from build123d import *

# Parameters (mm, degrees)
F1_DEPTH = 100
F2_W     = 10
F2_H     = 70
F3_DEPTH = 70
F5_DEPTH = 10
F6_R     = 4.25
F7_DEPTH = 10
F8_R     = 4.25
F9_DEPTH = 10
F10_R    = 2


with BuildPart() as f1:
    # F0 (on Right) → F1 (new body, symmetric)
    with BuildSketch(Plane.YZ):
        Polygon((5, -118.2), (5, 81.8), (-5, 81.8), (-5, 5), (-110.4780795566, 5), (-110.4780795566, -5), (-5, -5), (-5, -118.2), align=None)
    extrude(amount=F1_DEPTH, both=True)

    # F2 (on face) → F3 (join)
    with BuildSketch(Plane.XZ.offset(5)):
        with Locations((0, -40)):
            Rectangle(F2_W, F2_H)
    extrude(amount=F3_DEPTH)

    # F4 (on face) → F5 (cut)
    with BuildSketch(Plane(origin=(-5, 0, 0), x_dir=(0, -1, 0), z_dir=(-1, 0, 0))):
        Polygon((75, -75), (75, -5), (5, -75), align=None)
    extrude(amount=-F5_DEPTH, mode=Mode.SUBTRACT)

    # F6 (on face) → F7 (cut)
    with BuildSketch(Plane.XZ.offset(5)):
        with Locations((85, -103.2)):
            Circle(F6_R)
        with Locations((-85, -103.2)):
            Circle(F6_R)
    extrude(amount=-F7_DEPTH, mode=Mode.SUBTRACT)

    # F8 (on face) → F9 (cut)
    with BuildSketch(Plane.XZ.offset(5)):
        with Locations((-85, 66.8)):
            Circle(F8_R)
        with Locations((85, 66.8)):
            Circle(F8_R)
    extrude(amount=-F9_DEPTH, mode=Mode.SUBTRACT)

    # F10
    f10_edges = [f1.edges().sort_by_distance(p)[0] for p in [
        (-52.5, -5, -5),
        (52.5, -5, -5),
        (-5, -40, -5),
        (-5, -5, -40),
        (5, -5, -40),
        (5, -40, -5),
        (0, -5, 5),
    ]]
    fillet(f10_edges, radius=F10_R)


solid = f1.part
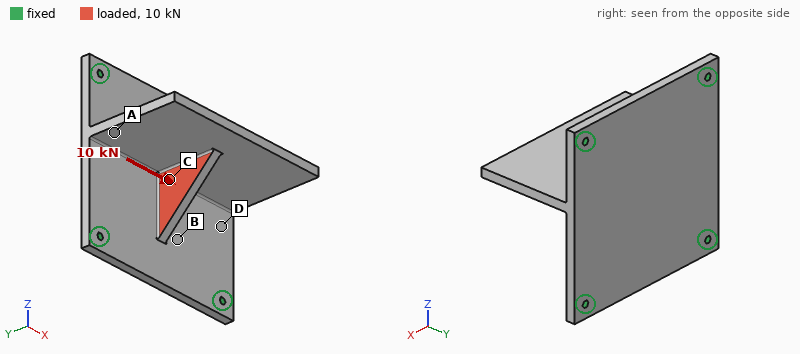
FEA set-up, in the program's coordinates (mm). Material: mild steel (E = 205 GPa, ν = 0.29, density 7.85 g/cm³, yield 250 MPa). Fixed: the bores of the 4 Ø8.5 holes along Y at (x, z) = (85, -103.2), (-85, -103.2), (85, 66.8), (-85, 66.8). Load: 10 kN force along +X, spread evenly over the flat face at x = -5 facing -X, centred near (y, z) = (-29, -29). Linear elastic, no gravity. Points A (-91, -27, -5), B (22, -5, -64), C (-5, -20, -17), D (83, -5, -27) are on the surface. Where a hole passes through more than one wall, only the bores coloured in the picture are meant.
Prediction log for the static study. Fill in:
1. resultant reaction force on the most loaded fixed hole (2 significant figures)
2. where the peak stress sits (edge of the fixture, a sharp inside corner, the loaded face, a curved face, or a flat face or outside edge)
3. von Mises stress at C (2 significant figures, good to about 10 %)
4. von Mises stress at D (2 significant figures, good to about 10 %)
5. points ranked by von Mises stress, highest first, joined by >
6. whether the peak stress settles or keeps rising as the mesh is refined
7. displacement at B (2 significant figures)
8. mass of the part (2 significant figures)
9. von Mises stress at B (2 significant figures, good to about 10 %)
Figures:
3.1 kN
edge of the fixture
32 MPa
13 MPa
C > B > D > A
keeps rising
9.6 µm
5.0 kg
19 MPa
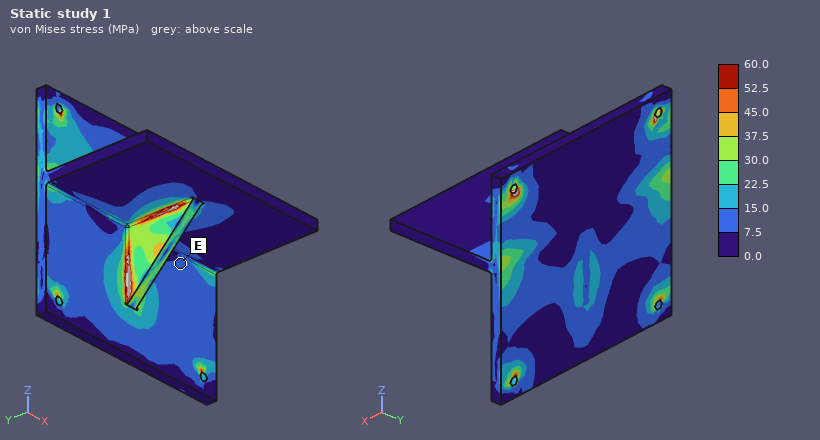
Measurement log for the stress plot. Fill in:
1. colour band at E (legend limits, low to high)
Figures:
7.5 to 15.0 MPa
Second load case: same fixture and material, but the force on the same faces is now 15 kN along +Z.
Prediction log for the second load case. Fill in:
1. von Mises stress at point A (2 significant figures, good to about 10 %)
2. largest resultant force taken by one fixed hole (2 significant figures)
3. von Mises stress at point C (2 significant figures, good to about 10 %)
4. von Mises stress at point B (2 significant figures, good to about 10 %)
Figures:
19 MPa
4.5 kN
32 MPa
40 MPa
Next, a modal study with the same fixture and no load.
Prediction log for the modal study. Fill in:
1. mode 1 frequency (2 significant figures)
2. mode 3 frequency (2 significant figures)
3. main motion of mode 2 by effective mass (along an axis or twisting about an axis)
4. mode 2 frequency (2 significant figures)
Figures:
890 Hz
970 Hz
along Y
920 Hz
